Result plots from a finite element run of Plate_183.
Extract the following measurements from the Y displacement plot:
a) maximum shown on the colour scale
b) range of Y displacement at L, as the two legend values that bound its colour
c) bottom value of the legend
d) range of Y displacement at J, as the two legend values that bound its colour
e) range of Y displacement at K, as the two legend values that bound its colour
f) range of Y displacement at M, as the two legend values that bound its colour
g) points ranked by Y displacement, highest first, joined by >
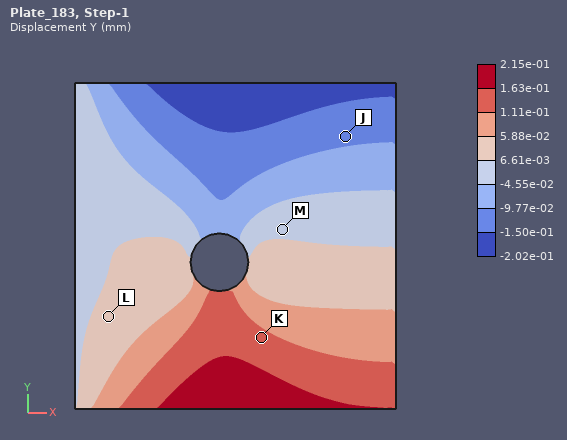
2.15e-01 mm
6.61e-03 to 5.88e-02 mm
-2.02e-01 mm
-1.50e-01 to -9.77e-02 mm
1.11e-01 to 1.63e-01 mm
-4.55e-02 to 6.61e-03 mm
K > L > M > J
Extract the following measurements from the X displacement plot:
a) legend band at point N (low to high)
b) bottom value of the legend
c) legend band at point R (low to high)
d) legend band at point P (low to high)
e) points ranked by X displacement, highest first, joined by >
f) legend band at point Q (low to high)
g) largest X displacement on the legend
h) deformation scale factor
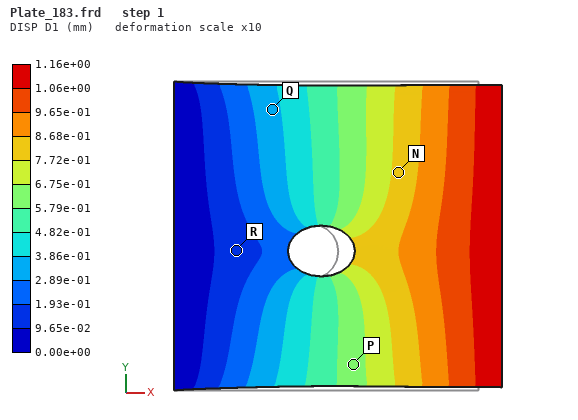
7.72e-01 to 8.68e-01 mm
0.00e+00 mm
9.65e-02 to 1.93e-01 mm
5.79e-01 to 6.75e-01 mm
N > P > Q > R
2.89e-01 to 3.86e-01 mm
1.16e+00 mm
10
